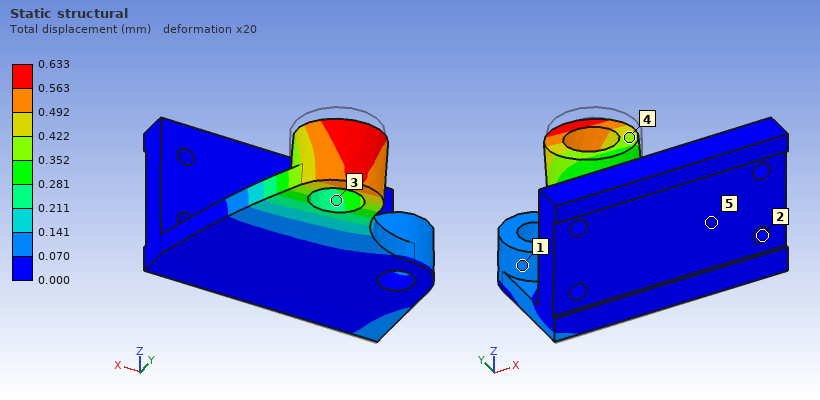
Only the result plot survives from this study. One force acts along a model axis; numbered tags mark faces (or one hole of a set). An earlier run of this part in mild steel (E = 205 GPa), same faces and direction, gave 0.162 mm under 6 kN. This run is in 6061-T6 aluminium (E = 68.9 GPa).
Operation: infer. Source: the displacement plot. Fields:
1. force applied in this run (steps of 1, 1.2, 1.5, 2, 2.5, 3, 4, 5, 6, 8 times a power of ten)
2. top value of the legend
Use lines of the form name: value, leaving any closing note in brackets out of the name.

force applied in this run: 8 kN
top value of the legend: 0.633 mm
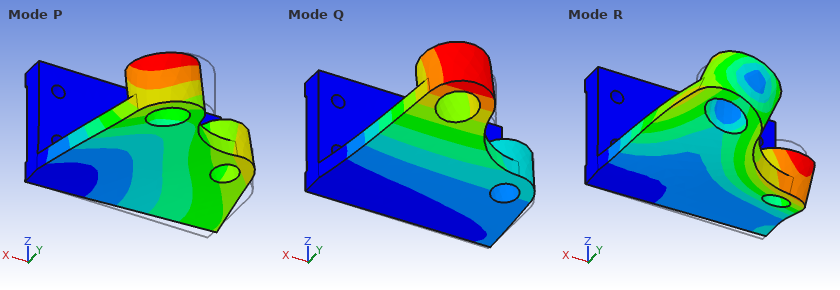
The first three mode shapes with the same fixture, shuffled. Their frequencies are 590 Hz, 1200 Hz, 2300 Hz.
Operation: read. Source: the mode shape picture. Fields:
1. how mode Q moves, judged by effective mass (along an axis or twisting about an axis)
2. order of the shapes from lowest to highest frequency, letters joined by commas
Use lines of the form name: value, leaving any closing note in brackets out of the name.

how mode Q moves, judged by effective mass: along Z
order of the shapes from lowest to highest frequency, letters joined by commas: Q, P, R
